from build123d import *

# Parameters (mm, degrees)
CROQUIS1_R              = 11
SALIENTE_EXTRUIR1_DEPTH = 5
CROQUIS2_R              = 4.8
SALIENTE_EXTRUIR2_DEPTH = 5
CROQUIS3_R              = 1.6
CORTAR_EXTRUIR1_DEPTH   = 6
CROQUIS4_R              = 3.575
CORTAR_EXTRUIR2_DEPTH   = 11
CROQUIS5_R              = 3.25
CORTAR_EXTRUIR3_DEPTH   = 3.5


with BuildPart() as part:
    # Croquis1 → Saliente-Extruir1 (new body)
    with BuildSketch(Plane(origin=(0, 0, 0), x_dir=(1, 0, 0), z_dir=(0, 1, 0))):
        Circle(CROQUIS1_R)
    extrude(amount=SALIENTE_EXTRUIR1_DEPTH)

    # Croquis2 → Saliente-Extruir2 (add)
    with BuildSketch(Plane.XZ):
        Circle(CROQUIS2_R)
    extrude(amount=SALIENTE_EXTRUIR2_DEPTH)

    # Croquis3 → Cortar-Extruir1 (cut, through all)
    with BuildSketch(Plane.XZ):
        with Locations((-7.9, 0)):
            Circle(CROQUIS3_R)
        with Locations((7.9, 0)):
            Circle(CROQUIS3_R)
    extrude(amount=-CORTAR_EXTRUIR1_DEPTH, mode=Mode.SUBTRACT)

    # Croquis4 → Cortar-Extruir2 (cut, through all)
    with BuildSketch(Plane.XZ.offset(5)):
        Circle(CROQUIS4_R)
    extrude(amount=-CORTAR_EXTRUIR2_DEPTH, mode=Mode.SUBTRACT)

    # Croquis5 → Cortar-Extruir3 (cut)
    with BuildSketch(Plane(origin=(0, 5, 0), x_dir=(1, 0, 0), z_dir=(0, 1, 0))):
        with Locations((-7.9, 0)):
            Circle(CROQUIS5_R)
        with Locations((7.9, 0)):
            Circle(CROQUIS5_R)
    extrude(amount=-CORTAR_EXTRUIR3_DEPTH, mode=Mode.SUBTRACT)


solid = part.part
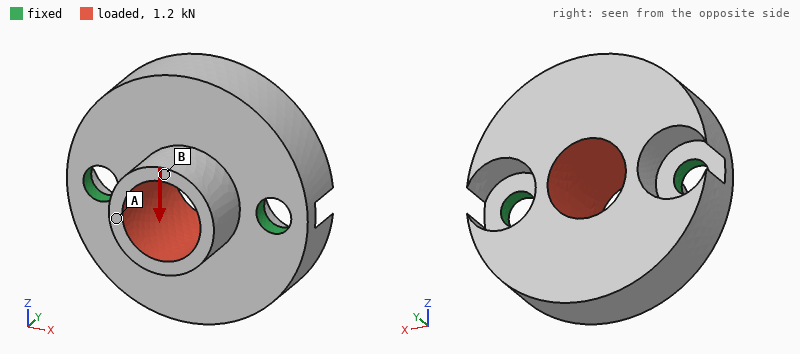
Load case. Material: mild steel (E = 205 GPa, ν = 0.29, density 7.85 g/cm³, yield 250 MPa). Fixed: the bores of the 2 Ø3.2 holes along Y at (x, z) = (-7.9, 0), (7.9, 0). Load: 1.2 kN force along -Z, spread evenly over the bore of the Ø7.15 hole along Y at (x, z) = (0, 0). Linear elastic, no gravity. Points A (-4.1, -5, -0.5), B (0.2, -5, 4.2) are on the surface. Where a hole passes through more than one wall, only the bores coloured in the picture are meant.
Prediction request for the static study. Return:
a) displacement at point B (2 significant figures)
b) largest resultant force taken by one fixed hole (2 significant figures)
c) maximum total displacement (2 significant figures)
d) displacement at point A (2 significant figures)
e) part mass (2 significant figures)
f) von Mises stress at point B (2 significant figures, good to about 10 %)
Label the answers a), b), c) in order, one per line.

a) 4.9 µm
b) 600 N
c) 5.0 µm
d) 4.1 µm
e) 13 g
f) 28 MPa
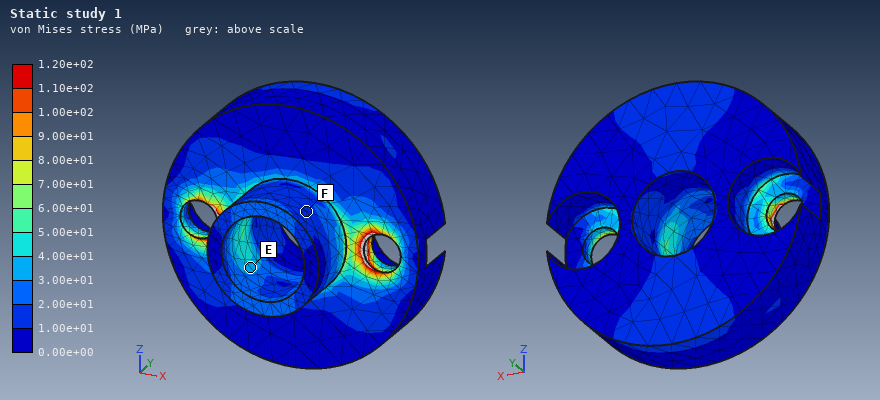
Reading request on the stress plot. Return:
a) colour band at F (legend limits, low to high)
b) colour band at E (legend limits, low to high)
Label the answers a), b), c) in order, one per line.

a) 1.00e+01 to 2.00e+01 MPa
b) 3.00e+01 to 4.00e+01 MPa
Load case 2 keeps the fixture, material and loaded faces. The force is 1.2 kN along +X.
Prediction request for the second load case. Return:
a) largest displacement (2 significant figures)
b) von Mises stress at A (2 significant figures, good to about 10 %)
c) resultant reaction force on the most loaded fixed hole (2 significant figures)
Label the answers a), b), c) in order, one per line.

a) 3.4 µm
b) 27 MPa
c) 610 N
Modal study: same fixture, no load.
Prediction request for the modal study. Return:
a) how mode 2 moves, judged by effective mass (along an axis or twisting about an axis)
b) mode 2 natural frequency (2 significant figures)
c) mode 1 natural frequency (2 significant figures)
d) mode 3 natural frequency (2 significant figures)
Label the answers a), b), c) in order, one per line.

a) along Y
b) 23 kHz
c) 10 kHz
d) 42 kHz
